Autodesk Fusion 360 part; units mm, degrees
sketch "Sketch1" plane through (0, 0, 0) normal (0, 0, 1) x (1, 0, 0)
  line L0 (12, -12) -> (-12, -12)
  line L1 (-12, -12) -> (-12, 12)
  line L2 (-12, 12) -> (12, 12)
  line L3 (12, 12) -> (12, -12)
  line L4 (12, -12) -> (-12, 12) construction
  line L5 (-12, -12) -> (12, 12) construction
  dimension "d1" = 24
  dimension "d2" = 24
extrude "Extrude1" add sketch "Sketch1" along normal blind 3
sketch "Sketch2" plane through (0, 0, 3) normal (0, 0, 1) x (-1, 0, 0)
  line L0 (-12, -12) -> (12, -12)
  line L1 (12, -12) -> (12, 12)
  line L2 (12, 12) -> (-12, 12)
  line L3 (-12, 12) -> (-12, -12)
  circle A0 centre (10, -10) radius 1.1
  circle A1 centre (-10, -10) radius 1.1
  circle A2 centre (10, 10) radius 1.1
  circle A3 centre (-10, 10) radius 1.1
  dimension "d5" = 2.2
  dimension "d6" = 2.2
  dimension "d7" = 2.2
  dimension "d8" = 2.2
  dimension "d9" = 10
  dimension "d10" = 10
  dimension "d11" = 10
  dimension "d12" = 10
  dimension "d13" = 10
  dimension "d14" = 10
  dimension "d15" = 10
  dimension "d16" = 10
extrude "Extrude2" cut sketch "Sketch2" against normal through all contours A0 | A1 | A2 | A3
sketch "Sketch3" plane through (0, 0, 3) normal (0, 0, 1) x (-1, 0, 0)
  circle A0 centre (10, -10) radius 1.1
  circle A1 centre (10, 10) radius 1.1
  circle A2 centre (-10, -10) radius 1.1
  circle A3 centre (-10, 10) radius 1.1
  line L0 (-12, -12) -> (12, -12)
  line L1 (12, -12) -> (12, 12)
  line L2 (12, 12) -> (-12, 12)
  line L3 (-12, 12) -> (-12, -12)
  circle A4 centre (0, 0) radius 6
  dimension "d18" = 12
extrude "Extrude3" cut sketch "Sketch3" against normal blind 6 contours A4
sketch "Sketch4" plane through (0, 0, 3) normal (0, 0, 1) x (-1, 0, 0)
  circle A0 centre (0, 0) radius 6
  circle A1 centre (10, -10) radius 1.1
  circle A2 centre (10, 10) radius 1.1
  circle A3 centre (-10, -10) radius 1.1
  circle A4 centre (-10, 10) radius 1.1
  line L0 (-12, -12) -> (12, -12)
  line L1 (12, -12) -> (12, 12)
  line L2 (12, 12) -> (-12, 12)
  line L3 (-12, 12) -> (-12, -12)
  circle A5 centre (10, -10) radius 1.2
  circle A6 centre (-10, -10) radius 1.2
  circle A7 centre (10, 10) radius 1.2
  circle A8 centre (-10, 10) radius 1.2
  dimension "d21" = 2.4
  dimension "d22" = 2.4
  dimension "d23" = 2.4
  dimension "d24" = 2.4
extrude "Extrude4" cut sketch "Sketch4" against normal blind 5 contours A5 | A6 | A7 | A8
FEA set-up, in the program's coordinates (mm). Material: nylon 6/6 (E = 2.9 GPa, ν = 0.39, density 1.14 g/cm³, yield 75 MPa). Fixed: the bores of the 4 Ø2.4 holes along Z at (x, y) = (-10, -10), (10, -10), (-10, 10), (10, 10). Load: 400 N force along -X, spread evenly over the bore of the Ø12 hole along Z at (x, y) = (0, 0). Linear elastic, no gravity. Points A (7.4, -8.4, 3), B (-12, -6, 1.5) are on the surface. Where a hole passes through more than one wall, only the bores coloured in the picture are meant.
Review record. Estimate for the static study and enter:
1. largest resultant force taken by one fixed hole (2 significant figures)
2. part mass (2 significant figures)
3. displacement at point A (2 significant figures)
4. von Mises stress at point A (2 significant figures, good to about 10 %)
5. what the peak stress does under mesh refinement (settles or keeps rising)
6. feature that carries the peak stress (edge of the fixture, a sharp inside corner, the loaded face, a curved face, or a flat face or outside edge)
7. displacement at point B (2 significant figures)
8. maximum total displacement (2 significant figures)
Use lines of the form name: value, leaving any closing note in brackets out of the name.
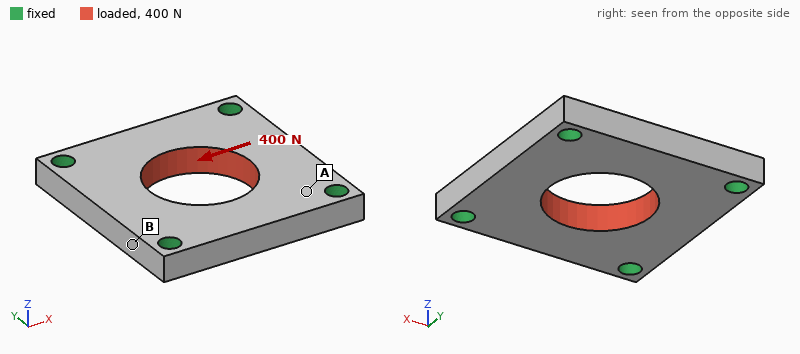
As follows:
largest resultant force taken by one fixed hole: 110 N
part mass: 1.5 g
displacement at point A: 6.7 µm
von Mises stress at point A: 6.3 MPa
what the peak stress does under mesh refinement: keeps rising
feature that carries the peak stress: edge of the fixture
displacement at point B: 17 µm
maximum total displacement: 33 µm
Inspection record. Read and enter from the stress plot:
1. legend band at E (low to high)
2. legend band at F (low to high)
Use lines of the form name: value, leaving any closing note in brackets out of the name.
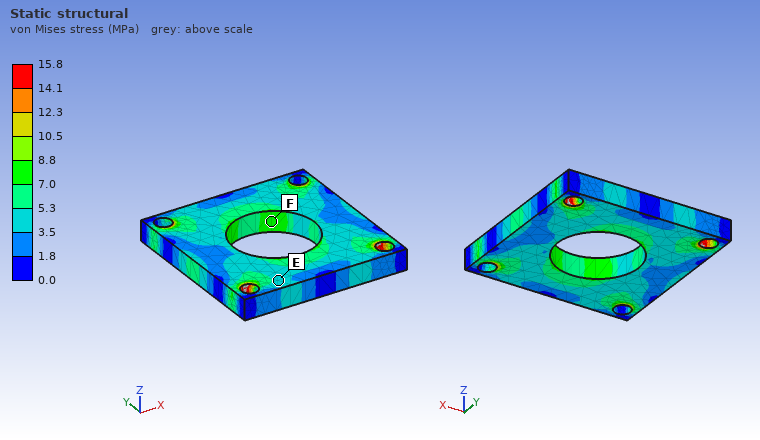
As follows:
legend band at E: 3.5 to 5.3 MPa
legend band at F: 7.0 to 8.8 MPa
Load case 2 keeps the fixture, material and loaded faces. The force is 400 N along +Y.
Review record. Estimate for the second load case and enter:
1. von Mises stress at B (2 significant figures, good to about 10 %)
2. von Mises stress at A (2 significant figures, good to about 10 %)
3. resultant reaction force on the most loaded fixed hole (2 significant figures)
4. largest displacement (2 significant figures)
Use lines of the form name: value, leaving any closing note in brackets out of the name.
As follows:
von Mises stress at B: 4.0 MPa
von Mises stress at A: 6.1 MPa
resultant reaction force on the most loaded fixed hole: 110 N
largest displacement: 33 µm
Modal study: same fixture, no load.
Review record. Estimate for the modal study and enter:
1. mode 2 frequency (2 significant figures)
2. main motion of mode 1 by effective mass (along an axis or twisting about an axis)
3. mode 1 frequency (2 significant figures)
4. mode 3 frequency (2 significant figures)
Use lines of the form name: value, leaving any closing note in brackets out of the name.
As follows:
mode 2 frequency: 12 kHz
main motion of mode 1 by effective mass: along Z
mode 1 frequency: 9700 Hz
mode 3 frequency: 12 kHz
